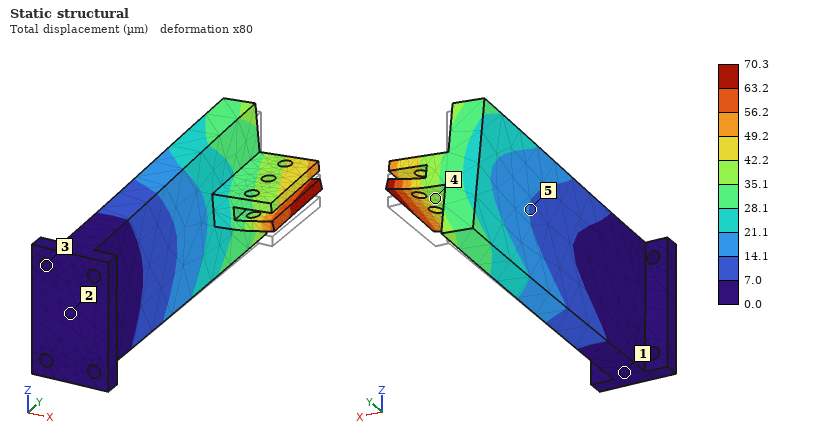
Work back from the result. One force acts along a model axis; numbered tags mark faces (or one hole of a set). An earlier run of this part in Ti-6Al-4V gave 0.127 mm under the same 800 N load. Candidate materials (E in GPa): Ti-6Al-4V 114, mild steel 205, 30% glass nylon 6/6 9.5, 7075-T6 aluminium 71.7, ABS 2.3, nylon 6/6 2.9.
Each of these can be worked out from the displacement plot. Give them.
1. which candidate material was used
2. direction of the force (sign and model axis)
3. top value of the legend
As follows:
mild steel
+Z
70.3 µm
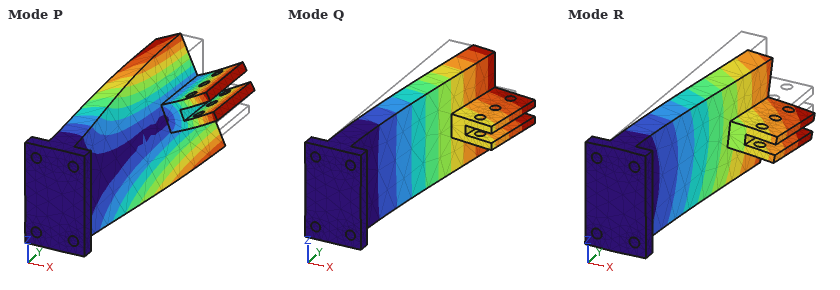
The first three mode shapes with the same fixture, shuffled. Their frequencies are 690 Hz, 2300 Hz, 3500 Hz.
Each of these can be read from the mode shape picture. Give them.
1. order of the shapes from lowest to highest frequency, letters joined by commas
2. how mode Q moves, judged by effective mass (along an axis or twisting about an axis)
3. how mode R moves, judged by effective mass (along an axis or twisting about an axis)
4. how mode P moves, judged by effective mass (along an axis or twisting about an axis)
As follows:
Q, R, P
along X
along Z
twisting about Y
